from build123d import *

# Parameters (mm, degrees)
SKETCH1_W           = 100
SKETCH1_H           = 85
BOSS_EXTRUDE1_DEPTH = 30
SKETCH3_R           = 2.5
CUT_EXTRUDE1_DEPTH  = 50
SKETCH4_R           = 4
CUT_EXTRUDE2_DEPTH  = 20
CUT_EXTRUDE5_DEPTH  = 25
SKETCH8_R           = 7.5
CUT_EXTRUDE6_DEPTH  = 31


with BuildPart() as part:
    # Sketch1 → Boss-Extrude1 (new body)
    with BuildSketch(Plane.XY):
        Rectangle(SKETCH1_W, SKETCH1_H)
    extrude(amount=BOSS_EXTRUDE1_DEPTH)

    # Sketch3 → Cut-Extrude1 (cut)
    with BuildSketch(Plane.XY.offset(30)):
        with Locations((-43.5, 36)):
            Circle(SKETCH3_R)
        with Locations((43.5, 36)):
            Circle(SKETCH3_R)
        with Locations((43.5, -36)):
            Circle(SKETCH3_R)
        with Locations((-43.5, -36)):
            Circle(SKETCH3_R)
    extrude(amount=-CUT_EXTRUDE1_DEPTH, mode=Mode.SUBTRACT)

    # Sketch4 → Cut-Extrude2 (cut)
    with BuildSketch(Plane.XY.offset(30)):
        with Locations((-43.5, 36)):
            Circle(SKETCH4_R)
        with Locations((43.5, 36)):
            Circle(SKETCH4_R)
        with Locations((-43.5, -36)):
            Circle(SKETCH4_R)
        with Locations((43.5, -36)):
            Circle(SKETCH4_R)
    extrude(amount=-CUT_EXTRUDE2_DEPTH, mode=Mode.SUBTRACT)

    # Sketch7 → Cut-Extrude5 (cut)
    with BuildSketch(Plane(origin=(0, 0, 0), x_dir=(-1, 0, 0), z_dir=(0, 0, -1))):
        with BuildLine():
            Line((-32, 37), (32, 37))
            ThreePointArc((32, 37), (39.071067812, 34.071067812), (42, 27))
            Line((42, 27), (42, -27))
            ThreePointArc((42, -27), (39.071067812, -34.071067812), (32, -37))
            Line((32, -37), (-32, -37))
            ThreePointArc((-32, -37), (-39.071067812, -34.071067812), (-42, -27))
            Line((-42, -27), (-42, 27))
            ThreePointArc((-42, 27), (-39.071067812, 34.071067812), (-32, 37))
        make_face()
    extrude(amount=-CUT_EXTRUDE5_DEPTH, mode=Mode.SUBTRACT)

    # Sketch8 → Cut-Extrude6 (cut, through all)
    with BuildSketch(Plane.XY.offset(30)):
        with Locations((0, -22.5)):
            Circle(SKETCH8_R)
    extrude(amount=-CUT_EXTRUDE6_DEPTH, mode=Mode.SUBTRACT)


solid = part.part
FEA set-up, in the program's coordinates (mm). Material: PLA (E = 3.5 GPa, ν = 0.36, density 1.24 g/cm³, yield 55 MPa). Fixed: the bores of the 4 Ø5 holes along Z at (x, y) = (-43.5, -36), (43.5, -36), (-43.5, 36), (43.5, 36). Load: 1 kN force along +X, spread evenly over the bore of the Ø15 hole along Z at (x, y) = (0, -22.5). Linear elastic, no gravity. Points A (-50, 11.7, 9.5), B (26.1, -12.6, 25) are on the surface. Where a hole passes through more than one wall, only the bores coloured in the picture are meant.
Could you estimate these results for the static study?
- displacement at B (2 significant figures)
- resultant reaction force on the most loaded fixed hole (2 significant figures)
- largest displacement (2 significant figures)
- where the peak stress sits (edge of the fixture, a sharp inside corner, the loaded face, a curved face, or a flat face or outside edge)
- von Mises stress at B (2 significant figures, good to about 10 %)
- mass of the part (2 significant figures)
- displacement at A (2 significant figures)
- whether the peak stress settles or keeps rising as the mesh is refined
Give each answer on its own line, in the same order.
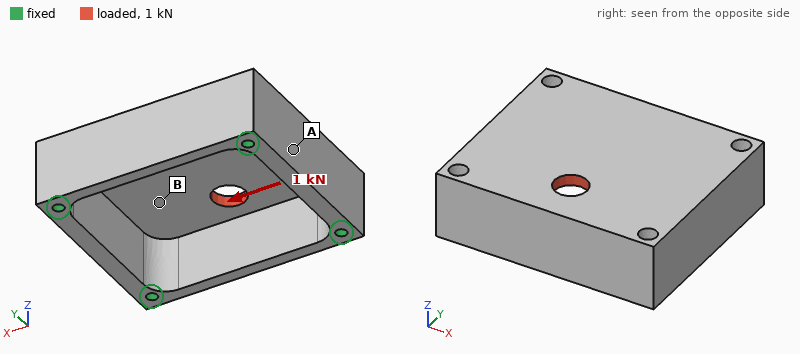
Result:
50 µm
370 N
68 µm
edge of the fixture
2.0 MPa
120 g
13 µm
keeps rising
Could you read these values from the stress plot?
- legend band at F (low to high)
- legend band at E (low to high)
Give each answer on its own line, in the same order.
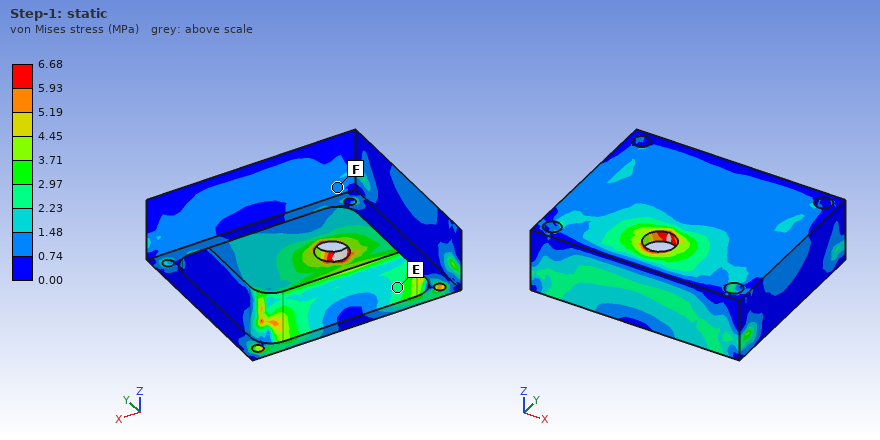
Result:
0.74 to 1.48 MPa
2.23 to 2.97 MPa
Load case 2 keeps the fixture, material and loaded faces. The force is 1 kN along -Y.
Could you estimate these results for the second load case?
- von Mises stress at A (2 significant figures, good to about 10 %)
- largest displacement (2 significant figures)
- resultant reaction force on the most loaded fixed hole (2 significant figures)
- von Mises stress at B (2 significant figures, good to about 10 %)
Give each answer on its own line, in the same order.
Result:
0.92 MPa
0.11 mm
290 N
2.9 MPa
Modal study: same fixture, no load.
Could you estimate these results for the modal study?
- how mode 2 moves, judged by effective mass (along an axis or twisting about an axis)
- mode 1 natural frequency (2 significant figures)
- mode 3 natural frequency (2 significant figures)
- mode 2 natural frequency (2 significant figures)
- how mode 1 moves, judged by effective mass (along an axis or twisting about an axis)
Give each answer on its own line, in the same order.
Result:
along Y
1600 Hz
2500 Hz
2200 Hz
along Z
